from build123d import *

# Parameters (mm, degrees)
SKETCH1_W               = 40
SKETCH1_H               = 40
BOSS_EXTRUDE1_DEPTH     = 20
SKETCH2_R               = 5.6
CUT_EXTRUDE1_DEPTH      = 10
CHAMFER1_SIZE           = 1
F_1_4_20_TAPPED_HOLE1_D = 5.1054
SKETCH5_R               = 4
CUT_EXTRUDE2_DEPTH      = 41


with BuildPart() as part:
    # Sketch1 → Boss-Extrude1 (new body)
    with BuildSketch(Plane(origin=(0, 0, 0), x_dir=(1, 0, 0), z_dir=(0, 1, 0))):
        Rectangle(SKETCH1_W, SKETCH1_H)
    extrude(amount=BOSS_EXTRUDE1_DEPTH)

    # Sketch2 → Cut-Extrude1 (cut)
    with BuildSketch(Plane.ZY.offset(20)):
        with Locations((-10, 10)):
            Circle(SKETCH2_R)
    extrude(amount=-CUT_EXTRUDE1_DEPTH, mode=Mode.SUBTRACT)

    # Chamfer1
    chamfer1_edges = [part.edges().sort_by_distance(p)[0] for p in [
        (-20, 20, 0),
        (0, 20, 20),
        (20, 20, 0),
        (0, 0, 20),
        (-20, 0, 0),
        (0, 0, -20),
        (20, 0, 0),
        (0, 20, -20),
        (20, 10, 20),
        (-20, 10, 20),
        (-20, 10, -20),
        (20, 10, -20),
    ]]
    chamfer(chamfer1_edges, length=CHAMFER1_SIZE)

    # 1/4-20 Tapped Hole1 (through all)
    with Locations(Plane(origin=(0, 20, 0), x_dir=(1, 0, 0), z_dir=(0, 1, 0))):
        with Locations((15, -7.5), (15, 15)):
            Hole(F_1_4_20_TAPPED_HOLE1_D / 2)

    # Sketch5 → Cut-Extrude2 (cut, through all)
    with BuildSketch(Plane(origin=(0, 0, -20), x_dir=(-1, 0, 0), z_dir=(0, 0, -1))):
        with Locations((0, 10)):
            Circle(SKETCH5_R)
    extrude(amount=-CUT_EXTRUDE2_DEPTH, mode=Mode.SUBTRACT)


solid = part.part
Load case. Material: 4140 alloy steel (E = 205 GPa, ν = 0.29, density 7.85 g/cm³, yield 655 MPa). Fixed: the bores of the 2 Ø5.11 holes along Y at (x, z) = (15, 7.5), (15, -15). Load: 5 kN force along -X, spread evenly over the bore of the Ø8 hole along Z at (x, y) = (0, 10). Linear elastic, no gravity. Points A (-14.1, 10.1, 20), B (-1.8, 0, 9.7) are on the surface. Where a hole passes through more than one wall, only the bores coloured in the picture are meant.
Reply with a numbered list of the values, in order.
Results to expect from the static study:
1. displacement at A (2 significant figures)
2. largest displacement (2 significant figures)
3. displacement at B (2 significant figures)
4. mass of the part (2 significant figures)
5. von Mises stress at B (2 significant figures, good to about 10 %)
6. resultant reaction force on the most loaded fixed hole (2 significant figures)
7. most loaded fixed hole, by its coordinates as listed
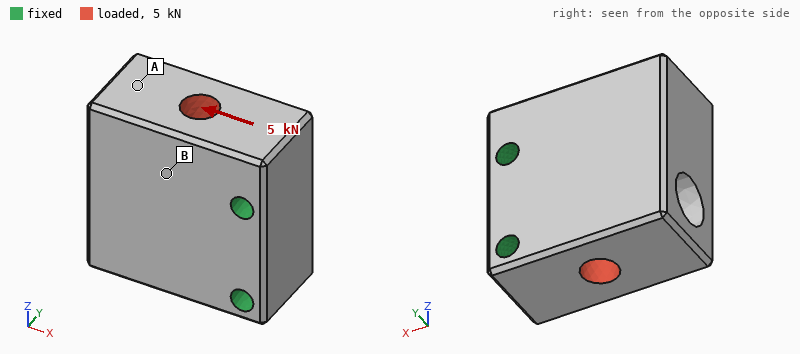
1. 1.0 µm
2. 1.1 µm
3. 0.73 µm
4. 220 g
5. 4.3 MPa
6. 3.2 kN
7. (15, 7.5)
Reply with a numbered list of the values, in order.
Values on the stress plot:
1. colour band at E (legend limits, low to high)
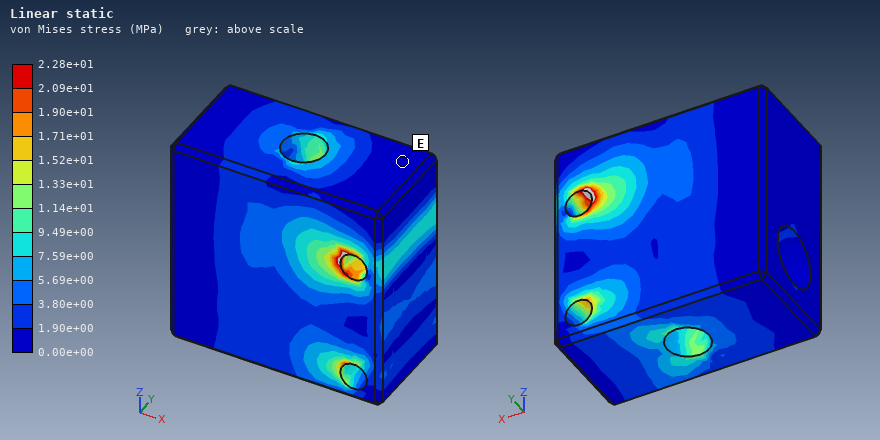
1. 0.00e+00 to 1.90e+00 MPa
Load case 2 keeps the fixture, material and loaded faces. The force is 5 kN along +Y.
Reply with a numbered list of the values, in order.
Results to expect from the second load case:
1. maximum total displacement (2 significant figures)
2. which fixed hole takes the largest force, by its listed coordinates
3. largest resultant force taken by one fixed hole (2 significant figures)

1. 6.9 µm
2. (15, 7.5)
3. 2.9 kN
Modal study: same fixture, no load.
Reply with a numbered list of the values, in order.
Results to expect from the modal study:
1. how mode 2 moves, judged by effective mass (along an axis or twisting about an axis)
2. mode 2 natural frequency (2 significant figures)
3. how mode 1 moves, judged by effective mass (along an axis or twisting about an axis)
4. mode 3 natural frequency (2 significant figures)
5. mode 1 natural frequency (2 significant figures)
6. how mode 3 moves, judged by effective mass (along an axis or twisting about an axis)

1. along Z
2. 14 kHz
3. along Y
4. 17 kHz
5. 9900 Hz
6. twisting about X
